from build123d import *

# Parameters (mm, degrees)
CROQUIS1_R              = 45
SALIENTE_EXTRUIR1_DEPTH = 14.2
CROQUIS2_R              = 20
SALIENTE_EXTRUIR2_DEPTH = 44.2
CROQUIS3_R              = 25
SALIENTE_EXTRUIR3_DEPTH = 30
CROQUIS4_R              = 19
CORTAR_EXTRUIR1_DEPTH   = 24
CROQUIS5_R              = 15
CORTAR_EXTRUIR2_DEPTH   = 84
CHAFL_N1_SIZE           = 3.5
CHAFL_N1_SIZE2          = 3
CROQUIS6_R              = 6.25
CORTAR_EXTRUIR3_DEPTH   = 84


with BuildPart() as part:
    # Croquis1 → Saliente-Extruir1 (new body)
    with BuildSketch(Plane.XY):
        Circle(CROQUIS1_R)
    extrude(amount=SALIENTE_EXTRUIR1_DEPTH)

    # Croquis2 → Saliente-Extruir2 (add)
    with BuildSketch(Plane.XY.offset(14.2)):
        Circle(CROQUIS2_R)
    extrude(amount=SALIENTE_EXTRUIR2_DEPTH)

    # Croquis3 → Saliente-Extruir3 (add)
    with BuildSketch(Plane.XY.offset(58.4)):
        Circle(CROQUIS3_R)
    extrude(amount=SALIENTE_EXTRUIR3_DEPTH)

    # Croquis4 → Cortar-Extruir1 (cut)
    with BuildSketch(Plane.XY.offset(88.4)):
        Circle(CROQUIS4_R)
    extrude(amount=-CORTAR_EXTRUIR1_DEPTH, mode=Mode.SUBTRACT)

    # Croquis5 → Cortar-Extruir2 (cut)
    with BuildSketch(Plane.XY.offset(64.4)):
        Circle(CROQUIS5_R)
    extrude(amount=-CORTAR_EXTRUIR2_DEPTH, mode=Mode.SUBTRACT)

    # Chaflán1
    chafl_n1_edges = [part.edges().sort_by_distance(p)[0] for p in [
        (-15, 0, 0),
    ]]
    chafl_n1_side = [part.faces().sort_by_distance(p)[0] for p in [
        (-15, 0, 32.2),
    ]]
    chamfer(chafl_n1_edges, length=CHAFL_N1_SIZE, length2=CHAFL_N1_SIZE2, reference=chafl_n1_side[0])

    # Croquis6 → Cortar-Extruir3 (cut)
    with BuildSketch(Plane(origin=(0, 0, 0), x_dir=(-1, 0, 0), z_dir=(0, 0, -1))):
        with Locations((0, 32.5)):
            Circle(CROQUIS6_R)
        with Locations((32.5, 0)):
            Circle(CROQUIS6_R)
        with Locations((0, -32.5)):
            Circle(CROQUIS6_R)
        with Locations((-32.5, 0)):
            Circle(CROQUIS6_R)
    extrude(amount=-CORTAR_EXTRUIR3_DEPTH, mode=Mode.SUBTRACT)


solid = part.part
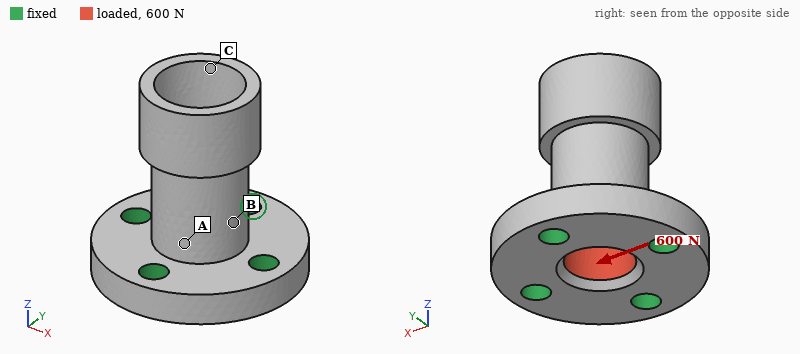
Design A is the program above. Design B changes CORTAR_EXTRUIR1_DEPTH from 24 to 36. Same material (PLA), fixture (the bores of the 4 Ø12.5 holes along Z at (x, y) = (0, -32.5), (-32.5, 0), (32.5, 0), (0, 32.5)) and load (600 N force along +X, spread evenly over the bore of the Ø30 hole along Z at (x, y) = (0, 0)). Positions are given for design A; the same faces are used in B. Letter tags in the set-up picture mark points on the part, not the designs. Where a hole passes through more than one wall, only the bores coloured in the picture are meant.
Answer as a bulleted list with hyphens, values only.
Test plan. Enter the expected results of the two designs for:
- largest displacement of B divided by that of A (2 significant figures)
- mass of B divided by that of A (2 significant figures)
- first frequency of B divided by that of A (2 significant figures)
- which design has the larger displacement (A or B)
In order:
- 0.68
- 0.96
- 0.96
- A
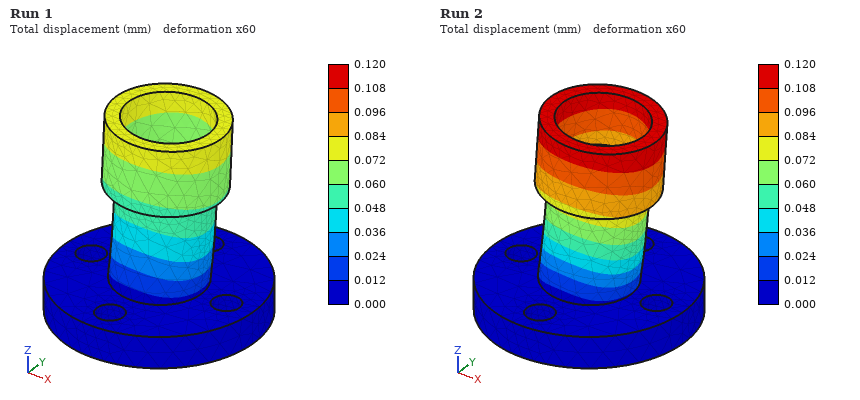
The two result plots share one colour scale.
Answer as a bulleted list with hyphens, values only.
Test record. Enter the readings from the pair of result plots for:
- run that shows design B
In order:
- Run 1
